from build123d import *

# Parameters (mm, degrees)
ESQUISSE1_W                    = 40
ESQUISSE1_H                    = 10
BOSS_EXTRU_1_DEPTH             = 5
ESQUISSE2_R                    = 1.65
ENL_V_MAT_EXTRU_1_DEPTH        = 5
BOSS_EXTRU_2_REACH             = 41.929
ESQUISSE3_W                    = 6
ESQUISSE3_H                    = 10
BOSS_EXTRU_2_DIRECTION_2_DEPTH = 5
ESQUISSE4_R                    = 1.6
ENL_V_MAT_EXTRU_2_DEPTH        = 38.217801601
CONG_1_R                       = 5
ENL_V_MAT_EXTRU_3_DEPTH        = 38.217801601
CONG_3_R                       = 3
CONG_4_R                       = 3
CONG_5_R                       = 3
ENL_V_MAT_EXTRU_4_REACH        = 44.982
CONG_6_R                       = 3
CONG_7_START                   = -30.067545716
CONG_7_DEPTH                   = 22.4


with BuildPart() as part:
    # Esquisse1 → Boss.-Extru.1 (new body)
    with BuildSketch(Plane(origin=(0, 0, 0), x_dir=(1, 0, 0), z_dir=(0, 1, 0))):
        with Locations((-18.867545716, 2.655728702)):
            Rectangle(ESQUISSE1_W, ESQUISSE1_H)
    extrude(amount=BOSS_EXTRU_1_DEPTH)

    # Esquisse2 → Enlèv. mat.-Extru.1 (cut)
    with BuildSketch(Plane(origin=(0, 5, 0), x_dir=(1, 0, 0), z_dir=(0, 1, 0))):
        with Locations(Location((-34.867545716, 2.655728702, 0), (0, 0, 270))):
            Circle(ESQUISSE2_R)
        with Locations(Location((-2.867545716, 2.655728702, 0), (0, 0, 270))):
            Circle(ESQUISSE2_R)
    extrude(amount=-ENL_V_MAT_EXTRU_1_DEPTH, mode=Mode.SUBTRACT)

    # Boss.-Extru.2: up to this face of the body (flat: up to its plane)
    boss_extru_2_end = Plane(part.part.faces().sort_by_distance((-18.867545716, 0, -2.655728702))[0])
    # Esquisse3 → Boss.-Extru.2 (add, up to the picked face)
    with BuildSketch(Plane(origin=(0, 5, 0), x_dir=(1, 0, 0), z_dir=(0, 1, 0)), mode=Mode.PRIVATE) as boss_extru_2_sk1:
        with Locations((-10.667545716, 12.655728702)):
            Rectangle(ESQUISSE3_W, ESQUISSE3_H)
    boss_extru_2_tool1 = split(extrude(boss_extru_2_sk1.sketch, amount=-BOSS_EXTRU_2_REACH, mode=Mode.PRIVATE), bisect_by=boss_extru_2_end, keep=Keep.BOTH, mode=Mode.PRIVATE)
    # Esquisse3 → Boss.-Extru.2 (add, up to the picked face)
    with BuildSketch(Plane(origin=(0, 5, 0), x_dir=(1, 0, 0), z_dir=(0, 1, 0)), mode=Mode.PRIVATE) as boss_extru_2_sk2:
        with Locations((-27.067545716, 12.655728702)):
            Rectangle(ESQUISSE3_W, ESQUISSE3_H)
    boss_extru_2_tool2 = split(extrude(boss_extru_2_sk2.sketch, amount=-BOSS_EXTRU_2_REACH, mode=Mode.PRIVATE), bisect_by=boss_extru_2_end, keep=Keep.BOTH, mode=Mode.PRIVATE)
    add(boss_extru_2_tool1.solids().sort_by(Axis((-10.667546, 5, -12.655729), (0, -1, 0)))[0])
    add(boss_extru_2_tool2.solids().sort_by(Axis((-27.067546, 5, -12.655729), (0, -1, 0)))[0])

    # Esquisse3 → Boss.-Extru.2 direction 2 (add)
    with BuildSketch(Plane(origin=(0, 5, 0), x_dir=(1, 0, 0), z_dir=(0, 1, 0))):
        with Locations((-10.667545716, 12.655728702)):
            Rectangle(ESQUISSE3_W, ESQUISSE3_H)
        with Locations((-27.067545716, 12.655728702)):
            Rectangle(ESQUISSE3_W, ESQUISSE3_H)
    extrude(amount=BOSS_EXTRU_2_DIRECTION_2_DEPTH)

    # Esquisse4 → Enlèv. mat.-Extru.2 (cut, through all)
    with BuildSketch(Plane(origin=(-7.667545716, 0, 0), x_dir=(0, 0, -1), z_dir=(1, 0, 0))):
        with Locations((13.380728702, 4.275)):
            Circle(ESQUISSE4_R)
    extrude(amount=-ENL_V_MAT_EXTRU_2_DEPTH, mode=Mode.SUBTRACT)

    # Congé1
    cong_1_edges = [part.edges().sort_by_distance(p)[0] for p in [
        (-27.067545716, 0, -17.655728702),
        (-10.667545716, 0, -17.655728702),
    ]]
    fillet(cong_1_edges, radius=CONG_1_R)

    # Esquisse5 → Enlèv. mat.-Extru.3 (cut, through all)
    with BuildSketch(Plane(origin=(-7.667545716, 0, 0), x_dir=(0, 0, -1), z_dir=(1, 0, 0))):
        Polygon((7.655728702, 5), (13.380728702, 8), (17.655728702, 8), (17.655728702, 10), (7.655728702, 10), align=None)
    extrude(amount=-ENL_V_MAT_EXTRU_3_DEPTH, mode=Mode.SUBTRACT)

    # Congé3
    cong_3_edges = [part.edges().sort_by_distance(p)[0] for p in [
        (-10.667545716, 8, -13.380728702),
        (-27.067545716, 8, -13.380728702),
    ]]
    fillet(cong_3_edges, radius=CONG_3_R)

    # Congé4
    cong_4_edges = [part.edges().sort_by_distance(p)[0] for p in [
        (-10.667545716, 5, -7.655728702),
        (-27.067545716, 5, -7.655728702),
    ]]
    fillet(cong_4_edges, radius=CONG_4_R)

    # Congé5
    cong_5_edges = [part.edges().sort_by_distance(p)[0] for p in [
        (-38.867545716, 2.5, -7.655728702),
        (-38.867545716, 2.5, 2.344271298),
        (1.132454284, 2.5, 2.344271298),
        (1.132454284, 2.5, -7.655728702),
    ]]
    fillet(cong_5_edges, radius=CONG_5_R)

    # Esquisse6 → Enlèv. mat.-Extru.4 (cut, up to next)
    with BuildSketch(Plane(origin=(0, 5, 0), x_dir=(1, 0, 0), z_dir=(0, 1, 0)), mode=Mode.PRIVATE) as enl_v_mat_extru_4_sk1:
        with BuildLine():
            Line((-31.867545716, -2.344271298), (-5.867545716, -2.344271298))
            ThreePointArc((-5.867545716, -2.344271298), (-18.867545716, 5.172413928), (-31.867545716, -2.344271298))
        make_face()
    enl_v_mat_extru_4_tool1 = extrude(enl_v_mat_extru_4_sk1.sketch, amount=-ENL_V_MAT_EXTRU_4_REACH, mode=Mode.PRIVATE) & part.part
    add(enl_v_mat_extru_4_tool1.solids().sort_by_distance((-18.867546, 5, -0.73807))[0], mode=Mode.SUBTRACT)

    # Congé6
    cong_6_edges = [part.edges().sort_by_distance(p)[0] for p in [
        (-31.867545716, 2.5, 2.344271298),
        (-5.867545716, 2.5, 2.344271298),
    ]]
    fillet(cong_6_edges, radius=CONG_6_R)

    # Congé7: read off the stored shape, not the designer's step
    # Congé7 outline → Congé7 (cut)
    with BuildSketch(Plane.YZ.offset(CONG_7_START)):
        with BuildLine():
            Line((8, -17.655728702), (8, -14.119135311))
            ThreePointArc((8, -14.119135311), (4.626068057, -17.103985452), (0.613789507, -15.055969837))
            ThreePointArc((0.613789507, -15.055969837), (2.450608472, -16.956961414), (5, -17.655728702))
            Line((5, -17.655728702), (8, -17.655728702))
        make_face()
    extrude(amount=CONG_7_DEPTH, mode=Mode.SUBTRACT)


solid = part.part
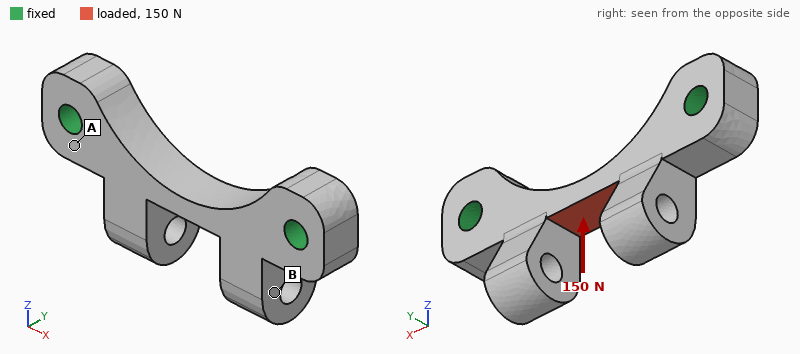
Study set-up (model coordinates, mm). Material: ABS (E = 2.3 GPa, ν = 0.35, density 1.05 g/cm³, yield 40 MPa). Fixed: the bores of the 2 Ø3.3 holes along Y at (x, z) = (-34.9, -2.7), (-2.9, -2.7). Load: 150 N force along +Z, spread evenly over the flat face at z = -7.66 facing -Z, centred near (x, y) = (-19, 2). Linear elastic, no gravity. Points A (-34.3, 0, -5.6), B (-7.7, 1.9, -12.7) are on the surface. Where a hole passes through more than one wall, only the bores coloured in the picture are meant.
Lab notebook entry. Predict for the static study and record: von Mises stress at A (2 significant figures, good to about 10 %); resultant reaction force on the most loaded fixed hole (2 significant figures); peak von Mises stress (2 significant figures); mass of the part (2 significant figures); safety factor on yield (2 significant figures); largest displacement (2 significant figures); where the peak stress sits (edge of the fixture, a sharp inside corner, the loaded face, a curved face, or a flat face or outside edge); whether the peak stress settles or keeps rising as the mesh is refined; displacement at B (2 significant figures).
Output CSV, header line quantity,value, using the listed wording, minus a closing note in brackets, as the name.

quantity,value
von Mises stress at A,4.4 MPa
resultant reaction force on the most loaded fixed hole,120 N
peak von Mises stress,24 MPa
mass of the part,1.9 g
safety factor on yield,1.7
largest displacement,0.19 mm
where the peak stress sits,the loaded face
whether the peak stress settles or keeps rising as the mesh is refined,settles
displacement at B,0.10 mm
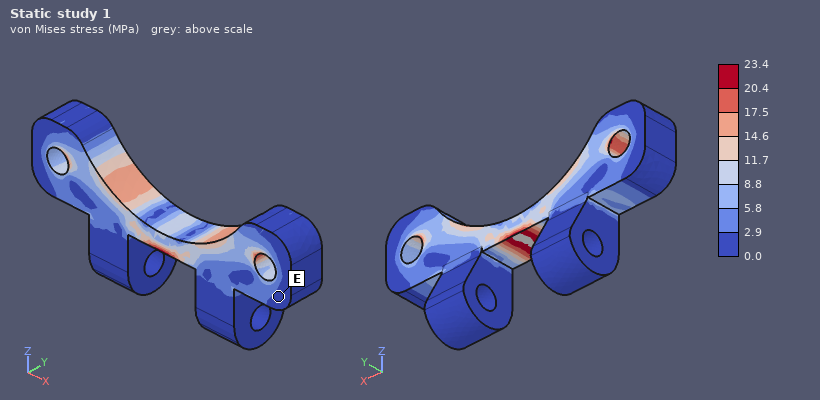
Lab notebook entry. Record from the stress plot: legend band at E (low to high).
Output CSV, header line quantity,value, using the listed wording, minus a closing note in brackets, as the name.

quantity,value
legend band at E,0.0 to 2.9 MPa
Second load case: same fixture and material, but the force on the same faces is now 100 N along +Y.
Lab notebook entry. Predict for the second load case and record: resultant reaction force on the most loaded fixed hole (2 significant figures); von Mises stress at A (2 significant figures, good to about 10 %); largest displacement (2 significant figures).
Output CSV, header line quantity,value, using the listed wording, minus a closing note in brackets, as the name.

quantity,value
resultant reaction force on the most loaded fixed hole,50 N
von Mises stress at A,8.0 MPa
largest displacement,0.20 mm
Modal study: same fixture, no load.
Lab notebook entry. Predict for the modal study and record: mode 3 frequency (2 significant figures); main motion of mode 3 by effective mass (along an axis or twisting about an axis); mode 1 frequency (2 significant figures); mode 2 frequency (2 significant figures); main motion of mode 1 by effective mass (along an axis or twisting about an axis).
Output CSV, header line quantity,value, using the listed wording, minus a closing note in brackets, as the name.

quantity,value
mode 3 frequency,5400 Hz
main motion of mode 3 by effective mass,along Z
mode 1 frequency,3800 Hz
mode 2 frequency,4400 Hz
main motion of mode 1 by effective mass,along Y
